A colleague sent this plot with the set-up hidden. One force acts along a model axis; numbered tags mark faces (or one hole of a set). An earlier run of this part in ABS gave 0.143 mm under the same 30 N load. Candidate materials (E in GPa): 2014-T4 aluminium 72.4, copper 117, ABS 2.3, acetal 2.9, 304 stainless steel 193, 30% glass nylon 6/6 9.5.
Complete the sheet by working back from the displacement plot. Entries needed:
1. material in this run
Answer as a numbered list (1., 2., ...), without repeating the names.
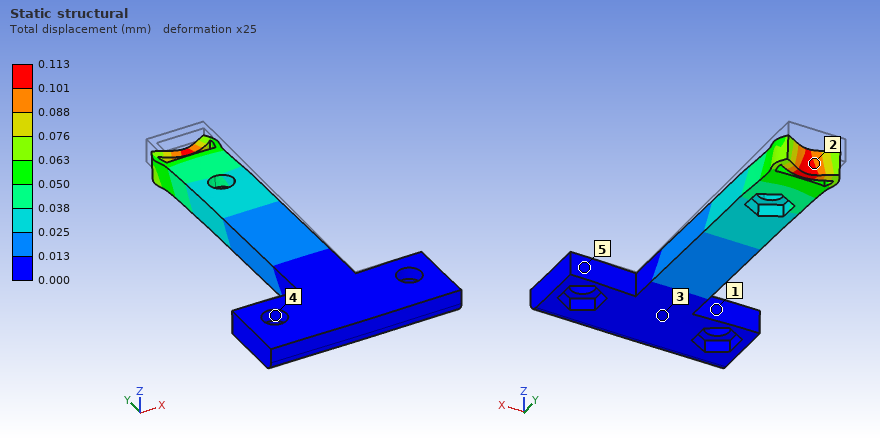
1. acetal
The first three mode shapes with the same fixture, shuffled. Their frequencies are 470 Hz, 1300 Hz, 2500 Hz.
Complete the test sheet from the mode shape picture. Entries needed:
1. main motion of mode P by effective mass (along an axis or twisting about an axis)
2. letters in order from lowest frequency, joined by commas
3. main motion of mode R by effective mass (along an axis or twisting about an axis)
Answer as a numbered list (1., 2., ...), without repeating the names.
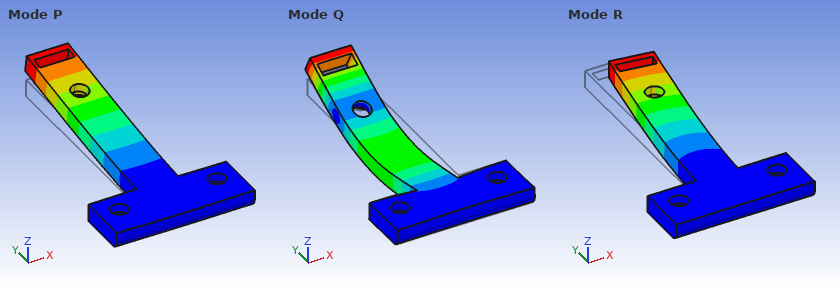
1. along Z
2. P, R, Q
3. along X
